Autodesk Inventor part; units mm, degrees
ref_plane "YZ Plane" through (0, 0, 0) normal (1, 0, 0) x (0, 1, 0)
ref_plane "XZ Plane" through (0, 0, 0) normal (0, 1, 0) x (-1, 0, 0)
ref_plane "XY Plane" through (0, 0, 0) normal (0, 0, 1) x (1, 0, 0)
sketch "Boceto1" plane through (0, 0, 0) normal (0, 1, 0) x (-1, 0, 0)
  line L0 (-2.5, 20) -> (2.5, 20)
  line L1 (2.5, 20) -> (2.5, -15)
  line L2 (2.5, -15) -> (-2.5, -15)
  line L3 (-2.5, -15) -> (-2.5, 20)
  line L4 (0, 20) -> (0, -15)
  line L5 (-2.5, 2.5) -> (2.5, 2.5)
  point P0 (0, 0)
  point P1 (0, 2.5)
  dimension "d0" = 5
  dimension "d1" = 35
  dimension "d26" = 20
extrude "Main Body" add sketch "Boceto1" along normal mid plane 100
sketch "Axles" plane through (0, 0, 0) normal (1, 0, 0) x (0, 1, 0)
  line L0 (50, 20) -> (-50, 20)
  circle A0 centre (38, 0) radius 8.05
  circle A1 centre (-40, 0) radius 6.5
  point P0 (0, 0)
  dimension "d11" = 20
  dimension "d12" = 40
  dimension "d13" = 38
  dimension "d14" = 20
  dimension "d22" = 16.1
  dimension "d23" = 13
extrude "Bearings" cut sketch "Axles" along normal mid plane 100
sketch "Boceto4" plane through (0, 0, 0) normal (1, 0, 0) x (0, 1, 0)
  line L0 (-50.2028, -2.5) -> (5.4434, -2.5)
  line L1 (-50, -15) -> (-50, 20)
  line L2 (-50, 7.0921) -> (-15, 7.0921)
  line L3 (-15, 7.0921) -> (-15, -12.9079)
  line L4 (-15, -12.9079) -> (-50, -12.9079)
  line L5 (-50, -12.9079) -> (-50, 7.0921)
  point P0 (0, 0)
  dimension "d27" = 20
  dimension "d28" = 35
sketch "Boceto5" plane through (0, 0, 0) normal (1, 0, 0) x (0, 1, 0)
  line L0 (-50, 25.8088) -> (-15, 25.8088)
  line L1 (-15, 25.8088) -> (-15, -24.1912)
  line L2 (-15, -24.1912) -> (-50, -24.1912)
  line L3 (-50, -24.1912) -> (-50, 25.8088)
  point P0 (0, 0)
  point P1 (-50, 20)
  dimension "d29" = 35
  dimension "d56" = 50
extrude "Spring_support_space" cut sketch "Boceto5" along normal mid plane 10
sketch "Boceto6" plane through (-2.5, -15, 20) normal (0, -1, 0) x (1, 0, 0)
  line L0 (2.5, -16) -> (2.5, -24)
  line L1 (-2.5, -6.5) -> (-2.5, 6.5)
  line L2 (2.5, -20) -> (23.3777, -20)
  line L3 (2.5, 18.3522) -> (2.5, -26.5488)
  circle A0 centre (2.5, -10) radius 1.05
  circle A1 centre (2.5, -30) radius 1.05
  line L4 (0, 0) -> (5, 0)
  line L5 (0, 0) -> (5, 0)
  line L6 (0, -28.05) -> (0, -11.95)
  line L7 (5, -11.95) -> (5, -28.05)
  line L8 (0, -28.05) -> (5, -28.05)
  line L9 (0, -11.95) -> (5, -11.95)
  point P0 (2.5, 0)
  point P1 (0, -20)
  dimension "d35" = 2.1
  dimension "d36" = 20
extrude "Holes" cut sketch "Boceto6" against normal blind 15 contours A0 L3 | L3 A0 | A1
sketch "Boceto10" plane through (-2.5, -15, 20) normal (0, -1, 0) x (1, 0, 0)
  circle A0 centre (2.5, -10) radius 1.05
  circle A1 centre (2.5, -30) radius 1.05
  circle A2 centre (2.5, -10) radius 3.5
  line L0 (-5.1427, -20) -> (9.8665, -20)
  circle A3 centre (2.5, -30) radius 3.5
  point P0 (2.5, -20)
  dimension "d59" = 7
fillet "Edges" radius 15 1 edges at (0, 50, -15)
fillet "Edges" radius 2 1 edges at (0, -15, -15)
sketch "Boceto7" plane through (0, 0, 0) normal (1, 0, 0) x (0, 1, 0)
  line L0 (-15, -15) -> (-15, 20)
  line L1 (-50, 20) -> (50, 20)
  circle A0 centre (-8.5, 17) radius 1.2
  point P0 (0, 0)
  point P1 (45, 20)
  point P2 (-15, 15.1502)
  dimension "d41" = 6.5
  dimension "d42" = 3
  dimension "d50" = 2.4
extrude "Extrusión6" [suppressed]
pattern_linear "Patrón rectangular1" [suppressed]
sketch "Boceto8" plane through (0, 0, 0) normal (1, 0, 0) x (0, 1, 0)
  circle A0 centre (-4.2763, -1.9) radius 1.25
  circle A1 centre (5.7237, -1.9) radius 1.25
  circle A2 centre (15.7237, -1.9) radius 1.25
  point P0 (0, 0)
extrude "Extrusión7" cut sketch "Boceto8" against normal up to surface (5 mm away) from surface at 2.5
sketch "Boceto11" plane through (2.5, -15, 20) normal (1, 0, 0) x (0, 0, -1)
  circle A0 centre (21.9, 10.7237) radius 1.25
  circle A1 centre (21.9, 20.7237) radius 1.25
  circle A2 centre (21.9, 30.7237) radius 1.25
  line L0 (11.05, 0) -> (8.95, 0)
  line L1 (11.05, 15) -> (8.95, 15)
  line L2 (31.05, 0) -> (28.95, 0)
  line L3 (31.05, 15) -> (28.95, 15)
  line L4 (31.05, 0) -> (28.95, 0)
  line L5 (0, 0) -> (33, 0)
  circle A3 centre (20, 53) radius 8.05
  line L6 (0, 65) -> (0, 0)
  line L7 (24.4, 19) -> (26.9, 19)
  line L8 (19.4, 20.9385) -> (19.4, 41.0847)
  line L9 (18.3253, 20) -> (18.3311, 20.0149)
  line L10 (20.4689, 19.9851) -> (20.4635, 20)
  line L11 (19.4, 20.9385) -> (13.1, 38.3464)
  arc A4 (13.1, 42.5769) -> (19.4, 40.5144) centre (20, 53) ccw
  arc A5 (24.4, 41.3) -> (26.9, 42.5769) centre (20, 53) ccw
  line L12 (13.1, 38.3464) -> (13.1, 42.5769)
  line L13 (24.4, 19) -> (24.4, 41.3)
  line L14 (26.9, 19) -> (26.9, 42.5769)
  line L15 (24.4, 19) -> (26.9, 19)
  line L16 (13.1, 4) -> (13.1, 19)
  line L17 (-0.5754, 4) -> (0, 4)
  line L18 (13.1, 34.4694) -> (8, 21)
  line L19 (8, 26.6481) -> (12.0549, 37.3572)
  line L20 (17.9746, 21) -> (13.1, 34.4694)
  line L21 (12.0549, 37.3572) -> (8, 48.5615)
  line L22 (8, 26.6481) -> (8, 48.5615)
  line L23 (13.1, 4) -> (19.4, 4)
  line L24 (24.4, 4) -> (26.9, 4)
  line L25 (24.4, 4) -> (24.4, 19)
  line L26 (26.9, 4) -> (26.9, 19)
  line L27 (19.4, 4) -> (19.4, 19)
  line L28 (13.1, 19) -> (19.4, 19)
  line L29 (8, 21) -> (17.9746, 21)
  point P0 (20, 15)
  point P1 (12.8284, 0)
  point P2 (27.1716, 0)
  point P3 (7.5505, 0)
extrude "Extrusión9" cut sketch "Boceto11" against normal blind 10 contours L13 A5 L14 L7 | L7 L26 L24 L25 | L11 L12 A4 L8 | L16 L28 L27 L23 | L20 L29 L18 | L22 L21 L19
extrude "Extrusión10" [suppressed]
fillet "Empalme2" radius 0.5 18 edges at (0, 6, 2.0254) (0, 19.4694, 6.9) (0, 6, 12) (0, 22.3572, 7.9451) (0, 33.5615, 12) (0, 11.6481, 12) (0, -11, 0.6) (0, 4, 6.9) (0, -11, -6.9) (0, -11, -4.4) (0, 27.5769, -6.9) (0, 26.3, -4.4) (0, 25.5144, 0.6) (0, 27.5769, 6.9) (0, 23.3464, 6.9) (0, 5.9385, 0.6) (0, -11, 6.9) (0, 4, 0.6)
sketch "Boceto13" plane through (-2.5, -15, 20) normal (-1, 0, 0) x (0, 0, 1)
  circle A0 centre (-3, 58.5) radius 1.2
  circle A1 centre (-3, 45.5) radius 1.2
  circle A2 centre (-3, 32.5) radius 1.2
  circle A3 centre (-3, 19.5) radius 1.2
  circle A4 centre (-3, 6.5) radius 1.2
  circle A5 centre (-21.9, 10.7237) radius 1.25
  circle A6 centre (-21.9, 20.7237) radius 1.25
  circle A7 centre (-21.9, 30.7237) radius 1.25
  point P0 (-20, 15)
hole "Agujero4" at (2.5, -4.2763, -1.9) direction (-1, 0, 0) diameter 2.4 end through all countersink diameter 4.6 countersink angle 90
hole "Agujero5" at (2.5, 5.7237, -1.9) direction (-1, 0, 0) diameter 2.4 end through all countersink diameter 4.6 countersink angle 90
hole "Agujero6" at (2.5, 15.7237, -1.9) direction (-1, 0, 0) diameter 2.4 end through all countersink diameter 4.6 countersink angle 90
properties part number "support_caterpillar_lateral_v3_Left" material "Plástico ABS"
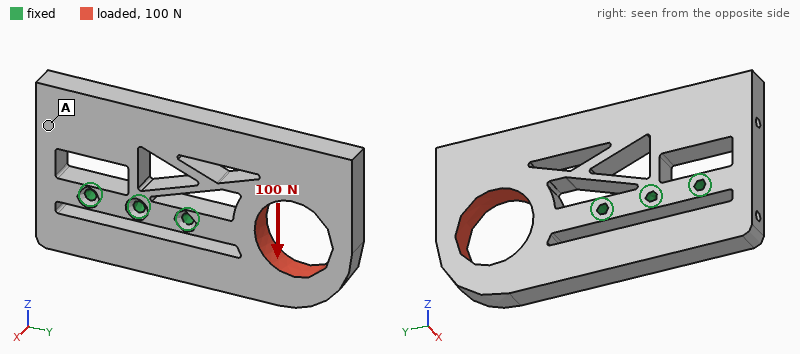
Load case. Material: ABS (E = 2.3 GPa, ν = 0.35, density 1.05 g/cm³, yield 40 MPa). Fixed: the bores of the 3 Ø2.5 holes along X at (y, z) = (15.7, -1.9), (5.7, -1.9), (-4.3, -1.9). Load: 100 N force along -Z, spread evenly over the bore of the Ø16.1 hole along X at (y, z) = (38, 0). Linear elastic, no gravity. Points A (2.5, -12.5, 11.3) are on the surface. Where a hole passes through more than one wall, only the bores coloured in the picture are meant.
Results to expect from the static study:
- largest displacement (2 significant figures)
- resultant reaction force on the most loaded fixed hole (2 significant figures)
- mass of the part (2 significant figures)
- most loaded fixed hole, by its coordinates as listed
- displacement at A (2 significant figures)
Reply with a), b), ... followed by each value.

a) 0.76 mm
b) 150 N
c) 8.5 g
d) (15.7, -1.9)
e) 0.24 mm
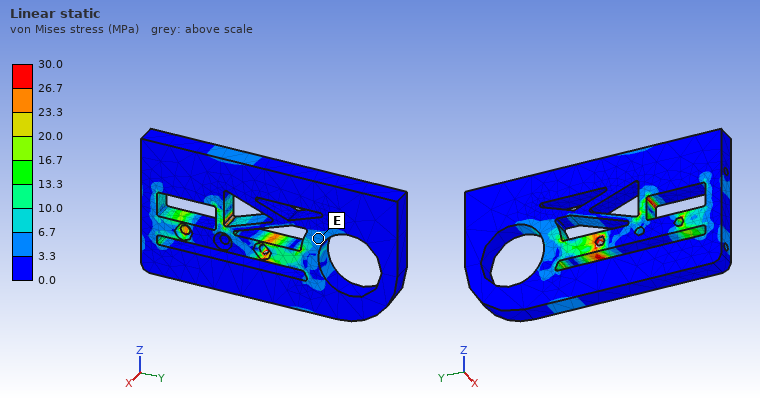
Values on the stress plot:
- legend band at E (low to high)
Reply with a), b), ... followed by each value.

a) 3.3 to 6.7 MPa
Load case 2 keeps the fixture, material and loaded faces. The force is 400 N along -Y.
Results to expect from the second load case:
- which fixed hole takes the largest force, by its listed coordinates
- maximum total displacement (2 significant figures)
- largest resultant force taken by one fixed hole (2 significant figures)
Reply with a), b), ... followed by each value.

a) (15.7, -1.9)
b) 0.21 mm
c) 230 N
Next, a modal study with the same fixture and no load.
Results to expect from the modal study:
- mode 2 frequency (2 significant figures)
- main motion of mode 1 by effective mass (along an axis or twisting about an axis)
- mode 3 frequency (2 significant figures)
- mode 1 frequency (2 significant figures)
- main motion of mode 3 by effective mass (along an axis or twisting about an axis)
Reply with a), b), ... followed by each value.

a) 870 Hz
b) along X
c) 1000 Hz
d) 590 Hz
e) along Z
